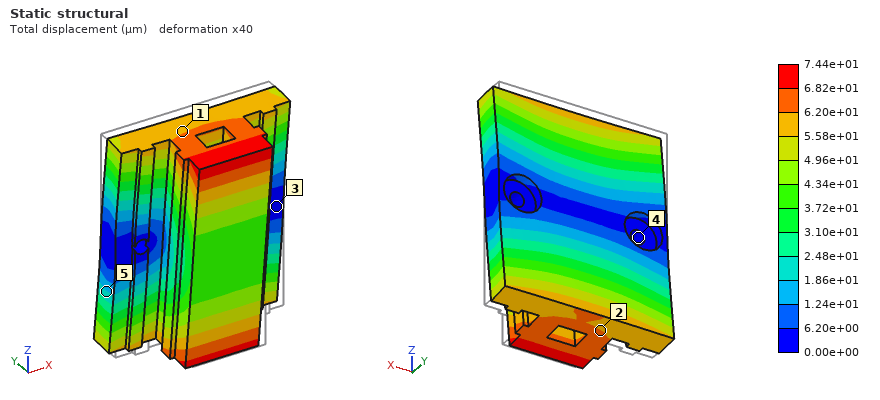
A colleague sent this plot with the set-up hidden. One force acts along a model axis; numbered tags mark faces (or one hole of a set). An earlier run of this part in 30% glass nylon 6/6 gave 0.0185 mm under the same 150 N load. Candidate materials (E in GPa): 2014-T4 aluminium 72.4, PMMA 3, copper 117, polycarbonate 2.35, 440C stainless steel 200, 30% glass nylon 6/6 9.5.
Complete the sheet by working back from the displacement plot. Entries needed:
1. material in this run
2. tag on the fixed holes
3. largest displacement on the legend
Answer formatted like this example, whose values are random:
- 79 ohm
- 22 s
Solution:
- polycarbonate
- 4
- 7.44e+01 µm
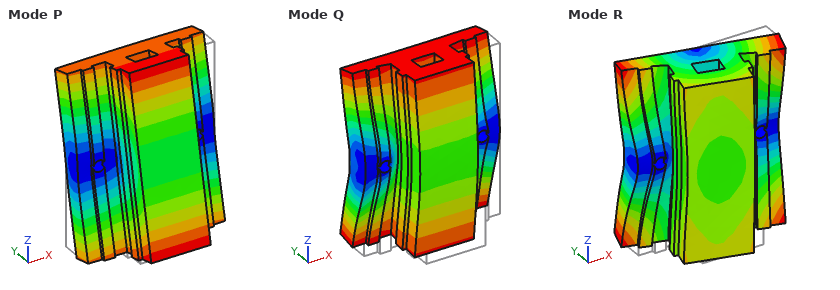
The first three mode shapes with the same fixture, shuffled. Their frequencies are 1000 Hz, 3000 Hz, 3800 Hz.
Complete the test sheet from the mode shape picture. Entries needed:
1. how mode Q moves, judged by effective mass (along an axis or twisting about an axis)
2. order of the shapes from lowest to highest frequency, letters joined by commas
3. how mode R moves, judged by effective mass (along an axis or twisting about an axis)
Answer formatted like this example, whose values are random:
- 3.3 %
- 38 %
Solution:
- along Y
- P, Q, R
- along X
